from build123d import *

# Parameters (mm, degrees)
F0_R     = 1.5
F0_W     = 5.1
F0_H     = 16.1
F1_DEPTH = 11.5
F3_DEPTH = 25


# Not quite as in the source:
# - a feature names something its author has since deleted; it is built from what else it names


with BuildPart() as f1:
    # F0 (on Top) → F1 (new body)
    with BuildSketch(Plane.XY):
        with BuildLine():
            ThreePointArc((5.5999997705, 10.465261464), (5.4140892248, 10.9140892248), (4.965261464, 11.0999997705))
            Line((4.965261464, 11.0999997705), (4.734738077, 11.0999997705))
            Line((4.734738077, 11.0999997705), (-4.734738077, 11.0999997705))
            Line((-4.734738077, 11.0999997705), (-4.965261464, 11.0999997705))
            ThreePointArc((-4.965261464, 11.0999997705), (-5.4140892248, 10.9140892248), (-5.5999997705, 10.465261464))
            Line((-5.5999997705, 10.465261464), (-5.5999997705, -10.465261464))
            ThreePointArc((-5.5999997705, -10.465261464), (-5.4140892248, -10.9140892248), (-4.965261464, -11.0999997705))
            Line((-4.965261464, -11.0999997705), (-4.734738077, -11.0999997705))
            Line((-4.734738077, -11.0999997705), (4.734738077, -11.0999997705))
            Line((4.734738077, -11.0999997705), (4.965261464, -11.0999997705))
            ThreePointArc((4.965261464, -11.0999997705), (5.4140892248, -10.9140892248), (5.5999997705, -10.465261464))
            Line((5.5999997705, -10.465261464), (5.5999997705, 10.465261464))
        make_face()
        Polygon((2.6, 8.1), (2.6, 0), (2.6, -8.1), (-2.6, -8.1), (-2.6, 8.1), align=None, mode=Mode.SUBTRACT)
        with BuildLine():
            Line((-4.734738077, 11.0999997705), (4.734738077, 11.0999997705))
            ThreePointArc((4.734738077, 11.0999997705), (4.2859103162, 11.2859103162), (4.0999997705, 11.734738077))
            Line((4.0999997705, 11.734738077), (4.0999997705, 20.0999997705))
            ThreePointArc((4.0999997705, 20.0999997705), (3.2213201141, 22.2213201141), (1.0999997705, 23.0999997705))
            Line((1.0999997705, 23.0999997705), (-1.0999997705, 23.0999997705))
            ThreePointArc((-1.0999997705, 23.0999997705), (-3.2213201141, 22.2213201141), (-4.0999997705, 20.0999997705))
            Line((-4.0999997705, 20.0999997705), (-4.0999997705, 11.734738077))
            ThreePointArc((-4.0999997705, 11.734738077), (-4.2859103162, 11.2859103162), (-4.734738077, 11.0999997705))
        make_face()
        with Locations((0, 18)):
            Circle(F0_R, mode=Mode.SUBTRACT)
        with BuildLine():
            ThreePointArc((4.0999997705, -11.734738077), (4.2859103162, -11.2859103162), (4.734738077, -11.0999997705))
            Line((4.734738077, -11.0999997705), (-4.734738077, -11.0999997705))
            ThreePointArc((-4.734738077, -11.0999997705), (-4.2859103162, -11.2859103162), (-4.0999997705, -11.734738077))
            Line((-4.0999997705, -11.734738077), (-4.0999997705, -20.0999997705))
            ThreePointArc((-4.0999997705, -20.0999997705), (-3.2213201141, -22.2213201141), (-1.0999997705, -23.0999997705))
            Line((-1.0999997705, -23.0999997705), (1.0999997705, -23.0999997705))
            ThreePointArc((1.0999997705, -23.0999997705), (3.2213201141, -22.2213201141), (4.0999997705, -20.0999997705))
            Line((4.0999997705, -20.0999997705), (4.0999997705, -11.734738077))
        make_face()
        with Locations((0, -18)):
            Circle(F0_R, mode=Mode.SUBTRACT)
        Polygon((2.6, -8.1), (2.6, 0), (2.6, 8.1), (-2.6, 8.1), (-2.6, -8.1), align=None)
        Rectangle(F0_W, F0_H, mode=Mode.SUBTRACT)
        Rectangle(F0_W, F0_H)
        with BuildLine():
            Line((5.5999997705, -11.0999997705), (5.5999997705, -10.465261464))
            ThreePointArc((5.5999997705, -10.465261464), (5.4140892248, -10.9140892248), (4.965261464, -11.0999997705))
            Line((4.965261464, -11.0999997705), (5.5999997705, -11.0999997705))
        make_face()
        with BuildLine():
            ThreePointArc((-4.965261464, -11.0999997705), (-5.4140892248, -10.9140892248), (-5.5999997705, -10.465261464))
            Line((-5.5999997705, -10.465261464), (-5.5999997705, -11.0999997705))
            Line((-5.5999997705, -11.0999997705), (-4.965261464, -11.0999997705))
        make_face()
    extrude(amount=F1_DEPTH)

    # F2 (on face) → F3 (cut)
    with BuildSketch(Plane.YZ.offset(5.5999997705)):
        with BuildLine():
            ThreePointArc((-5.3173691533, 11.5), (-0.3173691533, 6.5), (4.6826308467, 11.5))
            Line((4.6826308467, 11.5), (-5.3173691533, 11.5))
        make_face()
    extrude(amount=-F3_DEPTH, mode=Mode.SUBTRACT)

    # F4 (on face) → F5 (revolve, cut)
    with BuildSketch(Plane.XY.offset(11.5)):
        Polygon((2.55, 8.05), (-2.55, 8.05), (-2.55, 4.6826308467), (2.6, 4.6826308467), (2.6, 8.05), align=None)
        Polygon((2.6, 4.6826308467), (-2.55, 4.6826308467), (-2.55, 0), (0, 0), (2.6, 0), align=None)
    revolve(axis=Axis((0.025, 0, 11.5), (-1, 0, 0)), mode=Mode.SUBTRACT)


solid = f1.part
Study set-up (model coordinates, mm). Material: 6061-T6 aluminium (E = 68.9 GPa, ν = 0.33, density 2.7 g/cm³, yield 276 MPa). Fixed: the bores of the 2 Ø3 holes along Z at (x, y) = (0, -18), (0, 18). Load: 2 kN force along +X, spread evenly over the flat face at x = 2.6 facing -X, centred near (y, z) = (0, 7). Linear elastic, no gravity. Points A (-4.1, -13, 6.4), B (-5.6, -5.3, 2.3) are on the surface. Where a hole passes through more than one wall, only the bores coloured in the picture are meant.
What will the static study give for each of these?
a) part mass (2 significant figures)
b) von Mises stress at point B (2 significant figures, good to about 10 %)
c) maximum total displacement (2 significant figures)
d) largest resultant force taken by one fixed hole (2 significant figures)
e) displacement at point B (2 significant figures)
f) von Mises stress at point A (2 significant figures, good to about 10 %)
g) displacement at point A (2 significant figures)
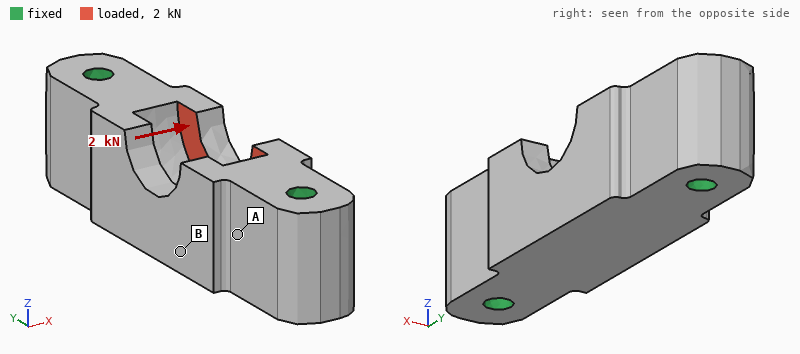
11 g
37 MPa
35 µm
1.0 kN
14 µm
14 MPa
6.9 µm
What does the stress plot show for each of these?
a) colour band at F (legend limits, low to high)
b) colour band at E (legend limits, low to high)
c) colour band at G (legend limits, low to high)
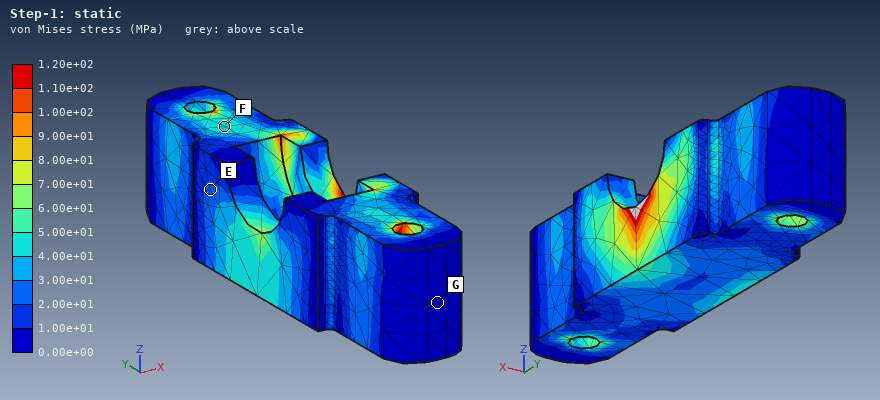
4.00e+01 to 5.00e+01 MPa
2.00e+01 to 3.00e+01 MPa
0.00e+00 to 1.00e+01 MPa
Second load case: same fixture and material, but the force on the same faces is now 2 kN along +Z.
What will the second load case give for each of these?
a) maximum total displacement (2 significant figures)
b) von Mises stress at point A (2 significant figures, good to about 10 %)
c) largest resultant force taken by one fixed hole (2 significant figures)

22 µm
12 MPa
1.2 kN
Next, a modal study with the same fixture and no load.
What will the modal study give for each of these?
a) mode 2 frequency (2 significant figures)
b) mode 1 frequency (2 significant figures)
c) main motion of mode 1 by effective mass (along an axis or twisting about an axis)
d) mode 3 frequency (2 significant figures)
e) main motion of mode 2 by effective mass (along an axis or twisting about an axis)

31 kHz
25 kHz
along X
40 kHz
along Z
